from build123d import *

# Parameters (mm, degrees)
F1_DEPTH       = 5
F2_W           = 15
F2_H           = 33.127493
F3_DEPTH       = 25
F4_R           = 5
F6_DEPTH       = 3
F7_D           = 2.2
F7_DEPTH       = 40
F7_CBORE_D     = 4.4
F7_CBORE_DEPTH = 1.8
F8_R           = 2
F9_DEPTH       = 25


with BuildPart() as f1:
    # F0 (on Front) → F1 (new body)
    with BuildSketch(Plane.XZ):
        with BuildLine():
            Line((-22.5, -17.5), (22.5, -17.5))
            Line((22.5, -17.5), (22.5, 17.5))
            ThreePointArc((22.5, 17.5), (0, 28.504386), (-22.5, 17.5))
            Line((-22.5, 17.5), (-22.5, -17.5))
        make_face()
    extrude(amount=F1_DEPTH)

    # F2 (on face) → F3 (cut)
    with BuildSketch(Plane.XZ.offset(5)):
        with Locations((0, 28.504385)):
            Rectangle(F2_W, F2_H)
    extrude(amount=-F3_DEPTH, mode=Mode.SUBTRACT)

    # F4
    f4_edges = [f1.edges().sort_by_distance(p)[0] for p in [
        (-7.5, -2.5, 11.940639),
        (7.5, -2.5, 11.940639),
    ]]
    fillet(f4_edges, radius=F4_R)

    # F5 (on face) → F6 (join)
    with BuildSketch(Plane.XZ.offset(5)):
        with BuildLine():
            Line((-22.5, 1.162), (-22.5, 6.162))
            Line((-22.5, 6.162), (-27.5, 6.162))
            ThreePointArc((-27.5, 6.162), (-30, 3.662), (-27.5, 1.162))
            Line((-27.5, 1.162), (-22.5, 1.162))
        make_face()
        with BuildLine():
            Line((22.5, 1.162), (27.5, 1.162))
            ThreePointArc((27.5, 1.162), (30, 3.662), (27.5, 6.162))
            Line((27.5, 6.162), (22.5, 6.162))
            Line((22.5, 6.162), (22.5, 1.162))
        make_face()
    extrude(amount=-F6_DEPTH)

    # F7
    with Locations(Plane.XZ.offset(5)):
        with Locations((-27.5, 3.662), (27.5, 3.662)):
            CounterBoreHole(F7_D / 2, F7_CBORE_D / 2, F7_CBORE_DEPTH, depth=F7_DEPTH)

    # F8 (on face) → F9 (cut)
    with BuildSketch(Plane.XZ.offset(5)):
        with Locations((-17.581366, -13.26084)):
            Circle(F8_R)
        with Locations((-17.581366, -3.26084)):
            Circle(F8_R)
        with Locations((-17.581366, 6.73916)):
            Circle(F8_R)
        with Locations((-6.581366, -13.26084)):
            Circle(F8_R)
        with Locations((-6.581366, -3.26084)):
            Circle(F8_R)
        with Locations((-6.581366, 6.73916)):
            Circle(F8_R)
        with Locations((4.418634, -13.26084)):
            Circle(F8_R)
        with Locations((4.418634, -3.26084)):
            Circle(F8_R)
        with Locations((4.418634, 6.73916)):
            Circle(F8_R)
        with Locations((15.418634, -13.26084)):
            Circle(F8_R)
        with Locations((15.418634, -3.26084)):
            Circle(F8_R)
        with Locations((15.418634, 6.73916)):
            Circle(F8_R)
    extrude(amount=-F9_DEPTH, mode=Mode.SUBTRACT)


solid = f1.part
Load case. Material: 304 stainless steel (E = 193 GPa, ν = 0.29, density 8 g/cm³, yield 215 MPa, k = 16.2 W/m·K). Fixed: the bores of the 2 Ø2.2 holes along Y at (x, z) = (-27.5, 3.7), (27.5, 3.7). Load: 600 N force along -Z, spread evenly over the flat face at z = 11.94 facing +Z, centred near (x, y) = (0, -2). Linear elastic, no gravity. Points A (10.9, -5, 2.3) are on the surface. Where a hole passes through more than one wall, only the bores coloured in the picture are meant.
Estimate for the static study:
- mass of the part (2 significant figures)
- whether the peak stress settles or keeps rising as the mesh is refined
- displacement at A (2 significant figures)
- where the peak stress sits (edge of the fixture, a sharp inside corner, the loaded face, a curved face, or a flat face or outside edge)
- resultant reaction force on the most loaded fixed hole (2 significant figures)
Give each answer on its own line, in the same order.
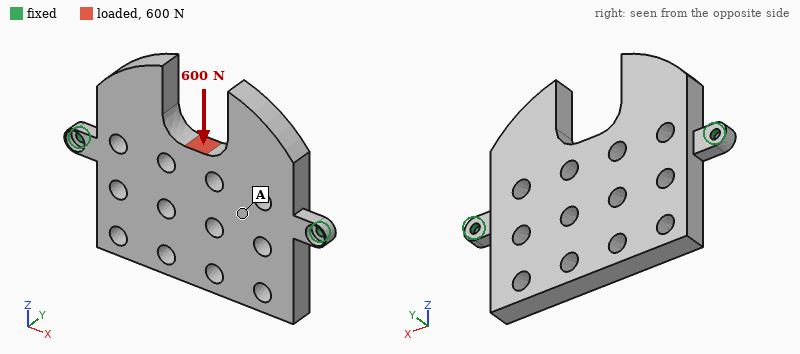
63 g
keeps rising
4.5 µm
edge of the fixture
300 N
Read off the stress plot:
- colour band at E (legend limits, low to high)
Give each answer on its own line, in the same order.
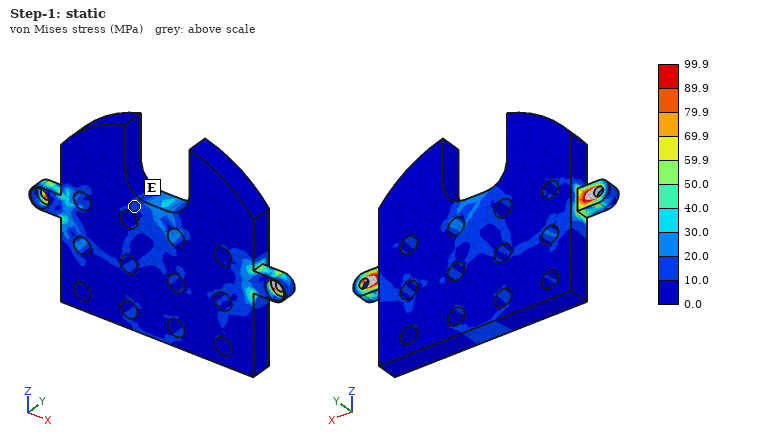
10.0 to 20.0 MPa
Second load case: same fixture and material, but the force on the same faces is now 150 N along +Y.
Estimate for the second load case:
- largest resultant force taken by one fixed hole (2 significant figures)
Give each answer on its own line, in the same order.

75 N
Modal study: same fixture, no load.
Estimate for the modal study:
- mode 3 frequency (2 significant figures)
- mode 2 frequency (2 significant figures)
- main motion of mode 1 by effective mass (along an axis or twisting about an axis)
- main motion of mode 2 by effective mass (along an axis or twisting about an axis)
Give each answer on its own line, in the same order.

5900 Hz
2900 Hz
twisting about X
along Y
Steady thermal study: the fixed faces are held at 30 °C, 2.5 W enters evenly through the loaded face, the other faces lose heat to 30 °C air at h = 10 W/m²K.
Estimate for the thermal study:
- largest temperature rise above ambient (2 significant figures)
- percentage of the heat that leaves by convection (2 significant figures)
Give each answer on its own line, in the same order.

54 K
50 %
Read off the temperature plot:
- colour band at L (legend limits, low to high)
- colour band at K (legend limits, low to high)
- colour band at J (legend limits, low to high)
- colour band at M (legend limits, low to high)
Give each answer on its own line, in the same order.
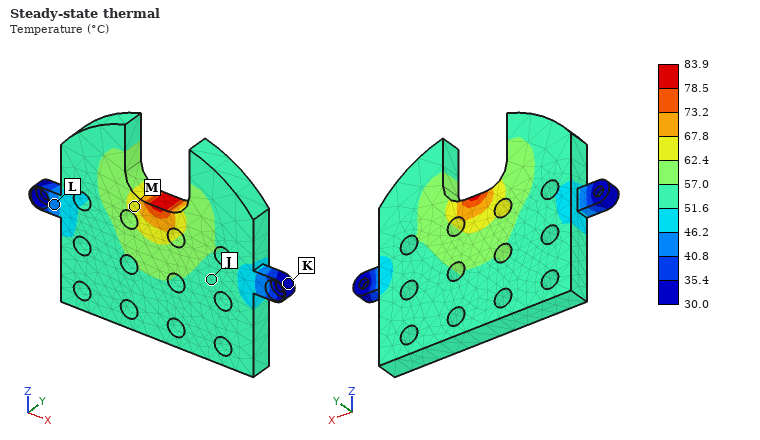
40.8 to 46.2 °C
30.0 to 35.4 °C
51.6 to 57.0 °C
62.4 to 67.8 °C
